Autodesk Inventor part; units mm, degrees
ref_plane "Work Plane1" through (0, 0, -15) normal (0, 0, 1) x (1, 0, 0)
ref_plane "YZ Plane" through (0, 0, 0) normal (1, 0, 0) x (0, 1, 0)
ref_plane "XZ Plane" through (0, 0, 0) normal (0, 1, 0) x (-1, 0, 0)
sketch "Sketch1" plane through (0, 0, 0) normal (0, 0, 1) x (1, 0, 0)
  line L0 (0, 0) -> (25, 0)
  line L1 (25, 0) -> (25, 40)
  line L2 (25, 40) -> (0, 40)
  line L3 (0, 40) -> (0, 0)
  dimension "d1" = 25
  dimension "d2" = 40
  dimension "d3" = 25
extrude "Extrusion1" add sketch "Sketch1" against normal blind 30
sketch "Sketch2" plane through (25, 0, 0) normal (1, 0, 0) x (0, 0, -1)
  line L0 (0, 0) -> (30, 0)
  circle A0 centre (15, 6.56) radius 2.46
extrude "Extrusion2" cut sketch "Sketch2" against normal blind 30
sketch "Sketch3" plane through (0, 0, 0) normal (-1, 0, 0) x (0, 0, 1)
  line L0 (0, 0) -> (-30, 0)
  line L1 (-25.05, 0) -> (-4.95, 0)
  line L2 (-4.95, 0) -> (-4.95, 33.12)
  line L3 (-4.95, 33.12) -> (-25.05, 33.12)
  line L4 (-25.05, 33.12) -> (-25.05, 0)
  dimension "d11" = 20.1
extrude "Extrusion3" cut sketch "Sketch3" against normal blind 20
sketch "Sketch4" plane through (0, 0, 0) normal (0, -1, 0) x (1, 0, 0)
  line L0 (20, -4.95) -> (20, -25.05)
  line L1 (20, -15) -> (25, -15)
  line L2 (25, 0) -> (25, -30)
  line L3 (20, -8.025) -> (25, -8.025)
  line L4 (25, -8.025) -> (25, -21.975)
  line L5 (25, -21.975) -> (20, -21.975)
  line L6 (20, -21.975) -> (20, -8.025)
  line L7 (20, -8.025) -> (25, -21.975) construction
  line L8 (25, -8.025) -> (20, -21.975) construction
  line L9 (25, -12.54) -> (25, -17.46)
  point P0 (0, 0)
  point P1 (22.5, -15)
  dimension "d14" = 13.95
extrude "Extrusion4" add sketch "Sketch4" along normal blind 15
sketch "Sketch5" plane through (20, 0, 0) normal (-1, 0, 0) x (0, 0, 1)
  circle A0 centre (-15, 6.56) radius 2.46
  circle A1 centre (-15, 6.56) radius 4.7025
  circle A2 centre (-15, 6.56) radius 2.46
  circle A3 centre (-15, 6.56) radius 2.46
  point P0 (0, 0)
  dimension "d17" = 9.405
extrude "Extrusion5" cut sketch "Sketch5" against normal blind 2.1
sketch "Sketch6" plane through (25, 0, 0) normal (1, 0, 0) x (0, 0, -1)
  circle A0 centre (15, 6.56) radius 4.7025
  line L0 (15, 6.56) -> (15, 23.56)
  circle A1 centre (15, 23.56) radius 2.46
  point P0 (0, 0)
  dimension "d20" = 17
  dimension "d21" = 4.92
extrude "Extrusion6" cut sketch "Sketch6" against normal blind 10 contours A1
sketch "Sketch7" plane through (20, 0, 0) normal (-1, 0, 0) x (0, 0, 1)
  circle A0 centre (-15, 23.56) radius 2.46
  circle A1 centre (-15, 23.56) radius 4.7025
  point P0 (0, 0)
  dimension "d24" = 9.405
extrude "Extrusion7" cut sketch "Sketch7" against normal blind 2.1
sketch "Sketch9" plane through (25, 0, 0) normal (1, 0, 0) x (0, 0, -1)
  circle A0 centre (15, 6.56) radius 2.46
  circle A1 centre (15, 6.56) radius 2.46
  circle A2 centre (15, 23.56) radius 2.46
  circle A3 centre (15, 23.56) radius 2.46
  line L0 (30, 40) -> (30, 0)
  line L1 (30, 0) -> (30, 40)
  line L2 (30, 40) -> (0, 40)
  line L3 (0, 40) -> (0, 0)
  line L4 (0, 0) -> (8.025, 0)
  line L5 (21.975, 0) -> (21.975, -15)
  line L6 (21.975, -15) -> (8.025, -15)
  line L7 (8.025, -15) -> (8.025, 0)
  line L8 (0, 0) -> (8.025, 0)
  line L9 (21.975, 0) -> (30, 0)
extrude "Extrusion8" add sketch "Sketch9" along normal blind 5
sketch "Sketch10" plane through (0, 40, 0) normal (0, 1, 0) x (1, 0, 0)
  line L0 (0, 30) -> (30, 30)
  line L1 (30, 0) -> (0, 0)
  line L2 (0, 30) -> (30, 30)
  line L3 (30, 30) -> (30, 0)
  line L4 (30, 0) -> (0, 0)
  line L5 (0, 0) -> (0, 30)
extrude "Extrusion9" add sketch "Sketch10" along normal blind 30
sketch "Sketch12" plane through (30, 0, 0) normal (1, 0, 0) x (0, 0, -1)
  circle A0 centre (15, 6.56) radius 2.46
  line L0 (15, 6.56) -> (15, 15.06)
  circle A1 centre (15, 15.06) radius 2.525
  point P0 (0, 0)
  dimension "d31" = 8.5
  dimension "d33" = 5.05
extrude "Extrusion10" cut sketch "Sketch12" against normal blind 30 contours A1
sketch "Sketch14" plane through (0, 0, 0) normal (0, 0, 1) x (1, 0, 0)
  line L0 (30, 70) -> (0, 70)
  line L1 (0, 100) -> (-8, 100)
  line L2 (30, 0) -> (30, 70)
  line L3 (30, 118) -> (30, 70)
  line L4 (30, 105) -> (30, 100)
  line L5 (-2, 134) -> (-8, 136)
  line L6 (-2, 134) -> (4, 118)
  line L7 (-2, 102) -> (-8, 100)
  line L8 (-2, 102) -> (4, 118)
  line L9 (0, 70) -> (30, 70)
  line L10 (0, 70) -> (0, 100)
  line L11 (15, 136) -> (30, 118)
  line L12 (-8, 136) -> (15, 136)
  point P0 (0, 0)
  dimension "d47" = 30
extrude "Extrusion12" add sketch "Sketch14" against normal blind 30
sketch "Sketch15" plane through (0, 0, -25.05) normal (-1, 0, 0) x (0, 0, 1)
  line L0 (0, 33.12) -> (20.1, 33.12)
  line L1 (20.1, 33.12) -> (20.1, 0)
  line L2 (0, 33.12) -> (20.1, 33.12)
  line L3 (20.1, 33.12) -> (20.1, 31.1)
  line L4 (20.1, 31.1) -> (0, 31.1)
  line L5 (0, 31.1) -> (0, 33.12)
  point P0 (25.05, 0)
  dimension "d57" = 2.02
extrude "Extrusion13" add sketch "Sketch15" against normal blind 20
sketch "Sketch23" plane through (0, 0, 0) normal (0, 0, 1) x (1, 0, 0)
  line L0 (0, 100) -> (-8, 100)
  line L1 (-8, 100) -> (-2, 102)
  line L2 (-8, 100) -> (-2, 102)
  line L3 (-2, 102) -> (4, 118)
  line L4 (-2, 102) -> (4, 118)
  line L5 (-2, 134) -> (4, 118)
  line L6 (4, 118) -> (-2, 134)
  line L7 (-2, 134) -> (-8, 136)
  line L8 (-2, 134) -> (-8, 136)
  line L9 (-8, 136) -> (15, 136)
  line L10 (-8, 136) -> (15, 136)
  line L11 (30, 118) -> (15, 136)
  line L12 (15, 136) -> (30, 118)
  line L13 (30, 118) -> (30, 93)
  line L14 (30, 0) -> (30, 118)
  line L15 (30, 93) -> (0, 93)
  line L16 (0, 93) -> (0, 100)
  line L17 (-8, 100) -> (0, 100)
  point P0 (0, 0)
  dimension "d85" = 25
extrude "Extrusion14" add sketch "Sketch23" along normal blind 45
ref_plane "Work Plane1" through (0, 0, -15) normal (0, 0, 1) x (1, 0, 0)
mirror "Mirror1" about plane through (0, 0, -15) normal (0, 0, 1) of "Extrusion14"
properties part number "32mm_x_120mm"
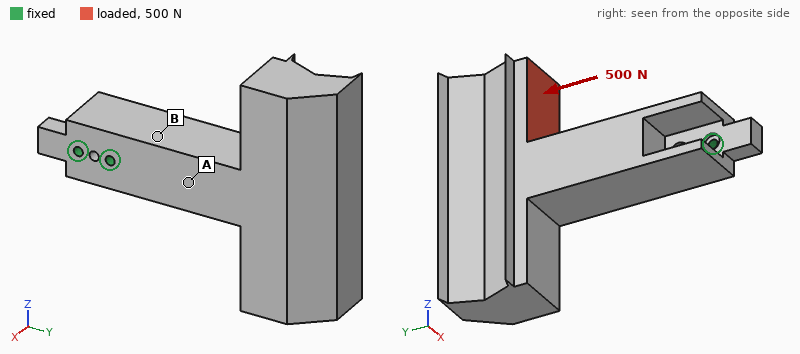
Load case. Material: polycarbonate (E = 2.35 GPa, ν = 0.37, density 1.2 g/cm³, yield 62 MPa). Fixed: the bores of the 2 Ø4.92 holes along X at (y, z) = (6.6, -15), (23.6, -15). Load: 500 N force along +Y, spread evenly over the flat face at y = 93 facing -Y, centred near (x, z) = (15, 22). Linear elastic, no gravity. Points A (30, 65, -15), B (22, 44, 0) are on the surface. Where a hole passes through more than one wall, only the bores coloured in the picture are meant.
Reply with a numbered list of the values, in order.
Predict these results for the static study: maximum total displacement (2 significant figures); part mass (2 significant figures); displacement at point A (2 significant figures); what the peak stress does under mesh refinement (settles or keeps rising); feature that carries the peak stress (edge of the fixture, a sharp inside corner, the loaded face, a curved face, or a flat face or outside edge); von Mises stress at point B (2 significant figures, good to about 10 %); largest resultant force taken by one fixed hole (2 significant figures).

1. 2.0 mm
2. 250 g
3. 0.46 mm
4. keeps rising
5. edge of the fixture
6. 6.1 MPa
7. 900 N
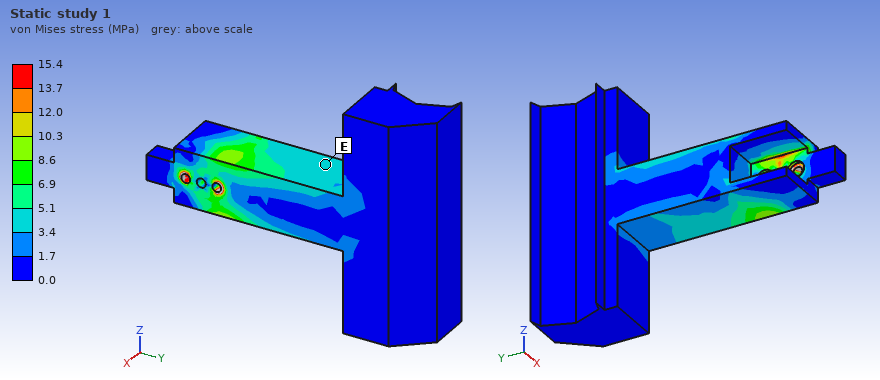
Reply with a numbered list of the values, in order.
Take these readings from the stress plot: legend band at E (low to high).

1. 3.4 to 5.1 MPa
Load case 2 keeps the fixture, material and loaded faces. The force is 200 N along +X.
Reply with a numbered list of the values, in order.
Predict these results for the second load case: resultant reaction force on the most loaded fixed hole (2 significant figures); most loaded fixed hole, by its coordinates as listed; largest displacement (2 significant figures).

1. 740 N
2. (23.6, -15)
3. 2.2 mm
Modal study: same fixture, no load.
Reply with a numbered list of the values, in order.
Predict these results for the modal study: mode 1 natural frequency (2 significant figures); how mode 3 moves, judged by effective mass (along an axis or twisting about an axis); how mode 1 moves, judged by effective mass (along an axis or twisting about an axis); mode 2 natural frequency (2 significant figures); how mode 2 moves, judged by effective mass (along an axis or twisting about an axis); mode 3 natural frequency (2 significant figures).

1. 140 Hz
2. twisting about Y
3. along X
4. 160 Hz
5. along Z
6. 240 Hz
